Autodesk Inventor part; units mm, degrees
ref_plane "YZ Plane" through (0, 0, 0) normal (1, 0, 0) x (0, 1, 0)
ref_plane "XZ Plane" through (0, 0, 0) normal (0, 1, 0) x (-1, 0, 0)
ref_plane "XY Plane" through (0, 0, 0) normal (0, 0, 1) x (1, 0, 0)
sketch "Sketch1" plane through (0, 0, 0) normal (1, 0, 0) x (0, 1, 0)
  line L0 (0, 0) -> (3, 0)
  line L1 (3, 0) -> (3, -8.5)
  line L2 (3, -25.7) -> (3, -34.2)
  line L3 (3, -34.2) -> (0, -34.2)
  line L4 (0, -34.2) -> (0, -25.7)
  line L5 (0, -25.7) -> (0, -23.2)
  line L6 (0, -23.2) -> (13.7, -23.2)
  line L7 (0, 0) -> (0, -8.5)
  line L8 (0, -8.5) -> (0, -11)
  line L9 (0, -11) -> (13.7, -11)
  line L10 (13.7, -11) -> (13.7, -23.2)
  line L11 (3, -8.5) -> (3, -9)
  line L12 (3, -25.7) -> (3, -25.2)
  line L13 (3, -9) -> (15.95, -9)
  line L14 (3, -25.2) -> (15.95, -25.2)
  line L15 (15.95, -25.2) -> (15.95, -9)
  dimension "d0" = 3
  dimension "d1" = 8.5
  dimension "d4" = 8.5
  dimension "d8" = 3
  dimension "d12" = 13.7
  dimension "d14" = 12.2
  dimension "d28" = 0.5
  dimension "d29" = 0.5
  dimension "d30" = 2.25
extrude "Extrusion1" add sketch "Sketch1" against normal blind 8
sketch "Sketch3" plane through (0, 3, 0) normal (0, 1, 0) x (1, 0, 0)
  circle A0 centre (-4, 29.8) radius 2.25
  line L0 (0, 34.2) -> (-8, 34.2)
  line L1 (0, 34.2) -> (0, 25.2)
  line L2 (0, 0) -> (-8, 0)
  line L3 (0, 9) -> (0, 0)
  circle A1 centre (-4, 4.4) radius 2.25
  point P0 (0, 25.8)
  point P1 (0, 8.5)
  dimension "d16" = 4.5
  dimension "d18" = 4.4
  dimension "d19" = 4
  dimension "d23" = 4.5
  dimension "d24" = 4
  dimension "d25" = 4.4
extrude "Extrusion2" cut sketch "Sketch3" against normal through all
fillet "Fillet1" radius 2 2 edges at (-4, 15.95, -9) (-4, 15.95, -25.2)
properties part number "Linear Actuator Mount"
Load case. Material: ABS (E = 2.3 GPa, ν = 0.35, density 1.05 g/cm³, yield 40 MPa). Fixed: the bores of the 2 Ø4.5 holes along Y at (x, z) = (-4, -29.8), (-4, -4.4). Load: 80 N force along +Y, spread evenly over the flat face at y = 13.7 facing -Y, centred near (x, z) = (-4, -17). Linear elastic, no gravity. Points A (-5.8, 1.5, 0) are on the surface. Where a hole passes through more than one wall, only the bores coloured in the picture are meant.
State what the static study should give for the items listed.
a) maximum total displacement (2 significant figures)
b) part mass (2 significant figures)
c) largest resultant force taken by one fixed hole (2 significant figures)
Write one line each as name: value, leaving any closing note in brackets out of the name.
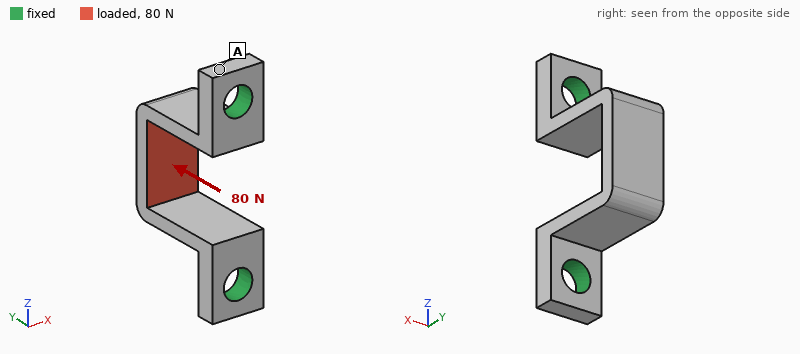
maximum total displacement: 0.13 mm
part mass: 1.1 g
largest resultant force taken by one fixed hole: 41 N
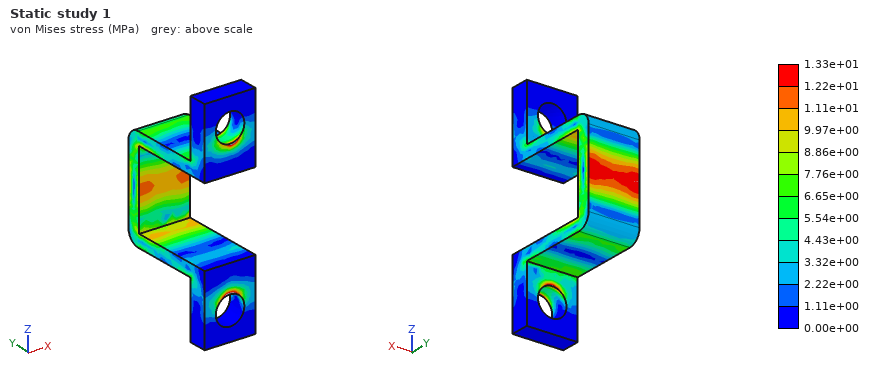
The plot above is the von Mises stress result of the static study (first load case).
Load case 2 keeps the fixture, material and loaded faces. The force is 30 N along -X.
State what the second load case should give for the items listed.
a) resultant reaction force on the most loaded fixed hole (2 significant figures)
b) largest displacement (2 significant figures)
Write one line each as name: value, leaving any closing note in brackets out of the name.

resultant reaction force on the most loaded fixed hole: 15 N
largest displacement: 0.23 mm
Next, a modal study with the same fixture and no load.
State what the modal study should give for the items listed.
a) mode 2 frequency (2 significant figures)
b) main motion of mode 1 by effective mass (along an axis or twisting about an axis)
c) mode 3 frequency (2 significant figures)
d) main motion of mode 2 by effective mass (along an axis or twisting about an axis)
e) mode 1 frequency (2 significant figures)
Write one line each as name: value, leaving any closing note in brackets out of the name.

mode 2 frequency: 2800 Hz
main motion of mode 1 by effective mass: along Z
mode 3 frequency: 4500 Hz
main motion of mode 2 by effective mass: along X
mode 1 frequency: 2500 Hz
